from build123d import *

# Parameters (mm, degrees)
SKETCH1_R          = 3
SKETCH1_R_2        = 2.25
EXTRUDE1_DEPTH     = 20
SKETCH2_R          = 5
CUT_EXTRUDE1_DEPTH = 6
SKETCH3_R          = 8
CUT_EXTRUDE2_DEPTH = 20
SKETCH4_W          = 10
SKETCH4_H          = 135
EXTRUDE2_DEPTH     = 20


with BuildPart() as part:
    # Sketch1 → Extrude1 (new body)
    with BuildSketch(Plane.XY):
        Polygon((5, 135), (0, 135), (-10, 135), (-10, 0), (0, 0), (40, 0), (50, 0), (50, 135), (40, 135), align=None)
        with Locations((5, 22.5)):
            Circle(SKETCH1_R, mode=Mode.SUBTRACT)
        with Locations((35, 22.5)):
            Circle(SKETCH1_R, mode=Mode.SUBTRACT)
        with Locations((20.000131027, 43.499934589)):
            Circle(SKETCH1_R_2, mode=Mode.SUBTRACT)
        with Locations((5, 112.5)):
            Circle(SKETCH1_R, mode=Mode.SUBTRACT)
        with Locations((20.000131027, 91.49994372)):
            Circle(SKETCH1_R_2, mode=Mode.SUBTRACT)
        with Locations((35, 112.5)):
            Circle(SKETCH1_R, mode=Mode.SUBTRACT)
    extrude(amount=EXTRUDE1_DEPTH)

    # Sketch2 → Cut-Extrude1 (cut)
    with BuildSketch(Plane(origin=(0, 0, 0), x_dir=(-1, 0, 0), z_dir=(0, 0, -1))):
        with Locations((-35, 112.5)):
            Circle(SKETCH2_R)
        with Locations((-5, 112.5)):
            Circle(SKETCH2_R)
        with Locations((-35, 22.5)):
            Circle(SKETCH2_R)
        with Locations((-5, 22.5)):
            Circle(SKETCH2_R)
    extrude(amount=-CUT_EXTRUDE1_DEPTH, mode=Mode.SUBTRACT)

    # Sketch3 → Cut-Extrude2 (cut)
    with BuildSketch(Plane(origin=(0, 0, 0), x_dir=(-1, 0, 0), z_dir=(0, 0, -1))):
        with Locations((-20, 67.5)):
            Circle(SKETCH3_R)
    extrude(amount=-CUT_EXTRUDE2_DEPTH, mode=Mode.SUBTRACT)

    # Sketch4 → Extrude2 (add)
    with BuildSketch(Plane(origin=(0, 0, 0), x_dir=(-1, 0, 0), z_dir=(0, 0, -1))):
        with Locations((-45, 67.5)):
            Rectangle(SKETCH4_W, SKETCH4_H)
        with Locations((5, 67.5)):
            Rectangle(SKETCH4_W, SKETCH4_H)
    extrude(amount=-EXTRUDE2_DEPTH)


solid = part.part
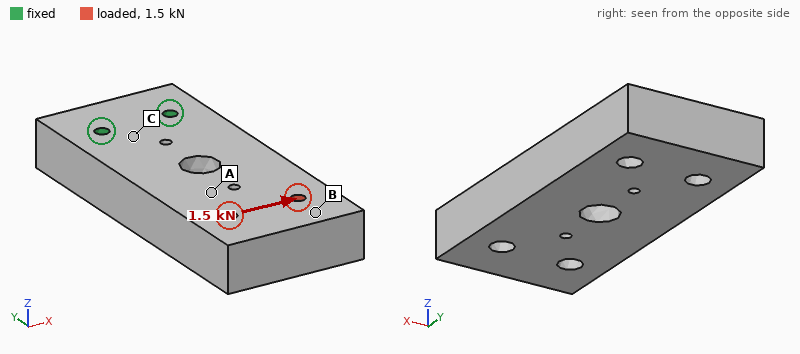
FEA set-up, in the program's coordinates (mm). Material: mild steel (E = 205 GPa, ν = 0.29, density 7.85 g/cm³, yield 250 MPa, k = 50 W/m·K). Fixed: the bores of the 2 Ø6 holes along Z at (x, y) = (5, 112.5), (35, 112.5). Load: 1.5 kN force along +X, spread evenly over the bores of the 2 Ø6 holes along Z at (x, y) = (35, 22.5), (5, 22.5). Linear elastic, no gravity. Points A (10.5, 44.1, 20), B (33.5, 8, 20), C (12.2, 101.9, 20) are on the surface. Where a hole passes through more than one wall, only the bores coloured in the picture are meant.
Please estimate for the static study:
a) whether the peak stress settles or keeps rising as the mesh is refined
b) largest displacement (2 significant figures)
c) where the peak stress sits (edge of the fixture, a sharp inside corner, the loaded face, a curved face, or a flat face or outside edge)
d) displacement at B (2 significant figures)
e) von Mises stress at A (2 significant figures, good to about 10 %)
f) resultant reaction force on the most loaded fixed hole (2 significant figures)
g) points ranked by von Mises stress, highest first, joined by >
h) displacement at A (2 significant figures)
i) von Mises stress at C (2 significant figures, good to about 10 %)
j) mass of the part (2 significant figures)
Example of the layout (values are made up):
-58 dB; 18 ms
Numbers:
keeps rising; 14 µm; edge of the fixture; 12 µm; 5.2 MPa; 4.1 kN; C > A > B; 7.7 µm; 8.9 MPa; 1.2 kg
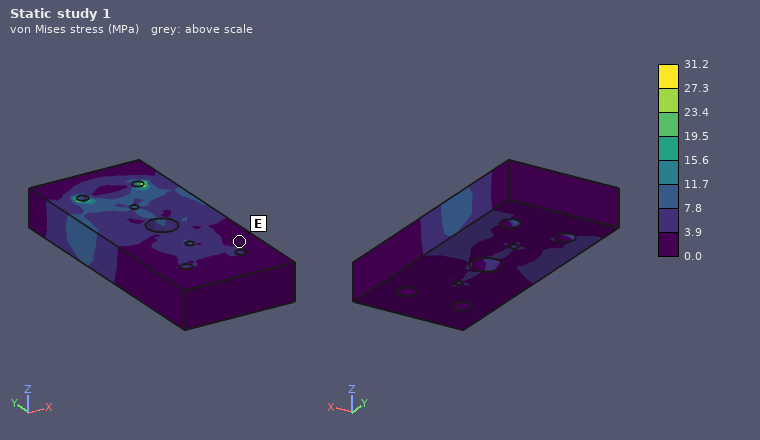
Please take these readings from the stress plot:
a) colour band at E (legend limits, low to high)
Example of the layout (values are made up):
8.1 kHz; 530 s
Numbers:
0.0 to 3.9 MPa
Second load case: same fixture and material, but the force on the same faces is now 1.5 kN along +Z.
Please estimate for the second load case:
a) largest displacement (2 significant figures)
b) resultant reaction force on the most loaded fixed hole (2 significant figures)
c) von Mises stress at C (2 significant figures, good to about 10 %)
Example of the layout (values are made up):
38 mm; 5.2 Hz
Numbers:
94 µm; 790 N; 30 MPa
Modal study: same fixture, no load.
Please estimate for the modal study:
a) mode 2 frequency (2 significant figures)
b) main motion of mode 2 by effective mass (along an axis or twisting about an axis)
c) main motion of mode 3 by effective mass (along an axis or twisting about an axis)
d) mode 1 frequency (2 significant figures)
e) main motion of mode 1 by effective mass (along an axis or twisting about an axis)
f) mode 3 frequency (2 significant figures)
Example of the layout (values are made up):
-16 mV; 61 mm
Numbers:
2700 Hz; along X; twisting about Y; 1000 Hz; along Z; 3900 Hz
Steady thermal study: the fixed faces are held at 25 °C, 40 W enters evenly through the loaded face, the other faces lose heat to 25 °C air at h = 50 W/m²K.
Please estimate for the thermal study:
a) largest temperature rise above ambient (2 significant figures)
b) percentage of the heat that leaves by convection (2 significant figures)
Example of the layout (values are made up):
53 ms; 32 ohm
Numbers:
42 K; 57 %
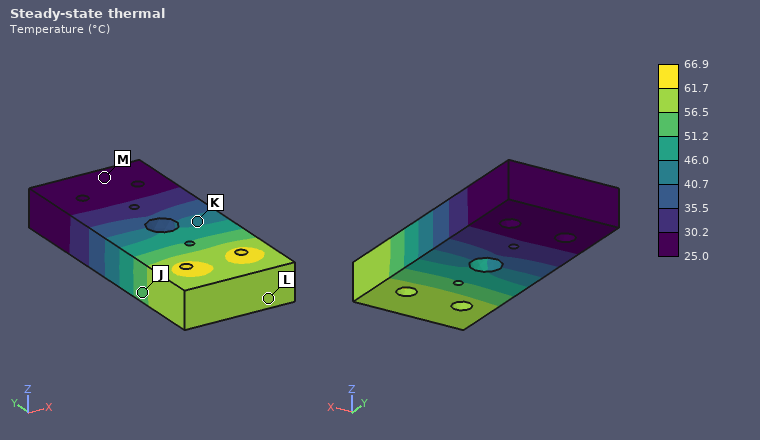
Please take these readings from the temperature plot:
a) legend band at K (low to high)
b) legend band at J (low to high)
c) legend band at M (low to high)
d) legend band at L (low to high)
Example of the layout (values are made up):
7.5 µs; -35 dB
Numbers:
40.7 to 46.0 °C; 51.2 to 56.5 °C; 25.0 to 30.2 °C; 56.5 to 61.7 °C
